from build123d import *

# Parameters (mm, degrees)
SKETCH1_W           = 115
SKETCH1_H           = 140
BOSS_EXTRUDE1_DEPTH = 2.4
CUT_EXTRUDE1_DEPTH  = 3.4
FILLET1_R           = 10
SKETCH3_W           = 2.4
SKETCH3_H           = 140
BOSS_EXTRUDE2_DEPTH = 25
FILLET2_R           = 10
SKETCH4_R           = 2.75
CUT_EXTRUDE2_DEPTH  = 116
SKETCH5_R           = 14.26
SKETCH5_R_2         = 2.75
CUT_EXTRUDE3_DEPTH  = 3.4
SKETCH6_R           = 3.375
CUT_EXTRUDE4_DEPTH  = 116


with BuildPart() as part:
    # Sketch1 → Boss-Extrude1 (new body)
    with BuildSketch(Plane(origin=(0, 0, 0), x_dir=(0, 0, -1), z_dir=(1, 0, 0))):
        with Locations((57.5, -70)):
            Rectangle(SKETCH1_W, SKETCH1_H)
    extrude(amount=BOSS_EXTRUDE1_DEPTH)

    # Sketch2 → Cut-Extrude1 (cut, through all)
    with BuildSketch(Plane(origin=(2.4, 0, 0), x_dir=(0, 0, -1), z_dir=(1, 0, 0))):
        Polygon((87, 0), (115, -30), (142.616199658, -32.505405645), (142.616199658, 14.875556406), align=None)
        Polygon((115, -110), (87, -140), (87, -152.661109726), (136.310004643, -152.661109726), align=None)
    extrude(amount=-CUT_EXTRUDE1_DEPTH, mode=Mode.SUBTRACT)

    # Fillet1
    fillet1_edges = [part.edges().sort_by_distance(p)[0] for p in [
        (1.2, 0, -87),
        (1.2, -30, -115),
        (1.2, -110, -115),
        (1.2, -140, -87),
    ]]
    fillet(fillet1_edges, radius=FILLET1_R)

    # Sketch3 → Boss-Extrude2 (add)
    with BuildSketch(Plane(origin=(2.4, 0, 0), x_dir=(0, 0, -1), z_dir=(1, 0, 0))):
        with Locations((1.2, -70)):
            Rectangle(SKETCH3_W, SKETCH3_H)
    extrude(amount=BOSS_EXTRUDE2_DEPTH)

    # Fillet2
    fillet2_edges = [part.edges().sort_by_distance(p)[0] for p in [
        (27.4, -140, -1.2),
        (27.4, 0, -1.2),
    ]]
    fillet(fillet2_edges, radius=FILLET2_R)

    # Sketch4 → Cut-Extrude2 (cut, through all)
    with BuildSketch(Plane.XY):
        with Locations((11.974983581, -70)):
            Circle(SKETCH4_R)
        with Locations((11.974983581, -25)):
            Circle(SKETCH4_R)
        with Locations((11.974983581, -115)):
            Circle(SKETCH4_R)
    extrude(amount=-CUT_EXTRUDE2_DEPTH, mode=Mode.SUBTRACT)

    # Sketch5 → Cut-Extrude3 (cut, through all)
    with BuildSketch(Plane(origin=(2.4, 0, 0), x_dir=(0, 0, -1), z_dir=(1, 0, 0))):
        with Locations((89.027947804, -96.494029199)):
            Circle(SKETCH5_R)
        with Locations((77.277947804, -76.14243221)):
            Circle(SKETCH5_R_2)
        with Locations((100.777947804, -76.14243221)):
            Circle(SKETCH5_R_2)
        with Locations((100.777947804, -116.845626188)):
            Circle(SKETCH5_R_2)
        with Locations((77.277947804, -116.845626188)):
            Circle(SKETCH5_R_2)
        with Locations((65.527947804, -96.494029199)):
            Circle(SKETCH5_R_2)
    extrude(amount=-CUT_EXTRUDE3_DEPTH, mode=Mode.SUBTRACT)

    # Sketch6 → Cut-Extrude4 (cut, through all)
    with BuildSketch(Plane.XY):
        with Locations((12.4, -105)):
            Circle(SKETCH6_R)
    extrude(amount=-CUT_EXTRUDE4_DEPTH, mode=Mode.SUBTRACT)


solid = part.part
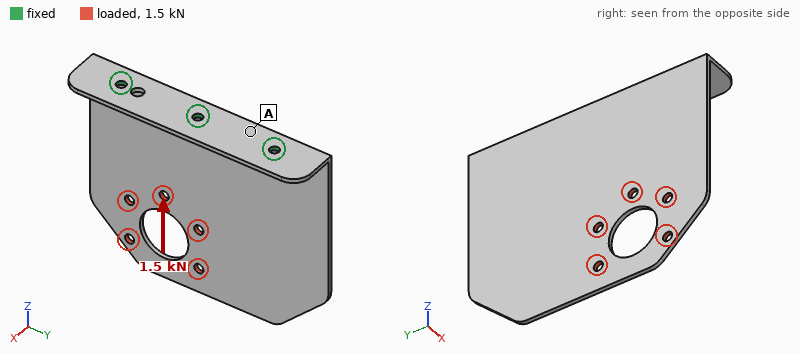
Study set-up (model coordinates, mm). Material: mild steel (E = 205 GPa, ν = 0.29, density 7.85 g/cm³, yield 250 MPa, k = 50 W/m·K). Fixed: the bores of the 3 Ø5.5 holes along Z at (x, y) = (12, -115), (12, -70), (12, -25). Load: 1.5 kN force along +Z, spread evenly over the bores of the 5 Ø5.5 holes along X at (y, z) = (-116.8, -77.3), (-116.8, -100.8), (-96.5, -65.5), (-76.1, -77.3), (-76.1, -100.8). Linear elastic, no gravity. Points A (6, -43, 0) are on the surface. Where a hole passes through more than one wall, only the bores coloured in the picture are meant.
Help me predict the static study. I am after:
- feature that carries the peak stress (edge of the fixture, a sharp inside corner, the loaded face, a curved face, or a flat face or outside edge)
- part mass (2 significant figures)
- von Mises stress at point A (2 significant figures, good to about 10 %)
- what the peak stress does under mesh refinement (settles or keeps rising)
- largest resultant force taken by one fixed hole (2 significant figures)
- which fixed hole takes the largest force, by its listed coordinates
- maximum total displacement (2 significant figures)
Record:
edge of the fixture
340 g
21 MPa
keeps rising
920 N
(12, -115)
0.40 mm
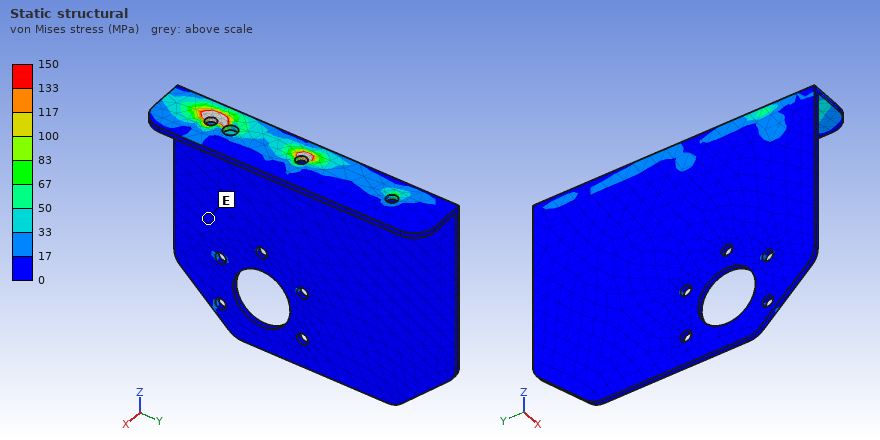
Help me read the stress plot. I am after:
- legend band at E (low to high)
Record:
0 to 17 MPa
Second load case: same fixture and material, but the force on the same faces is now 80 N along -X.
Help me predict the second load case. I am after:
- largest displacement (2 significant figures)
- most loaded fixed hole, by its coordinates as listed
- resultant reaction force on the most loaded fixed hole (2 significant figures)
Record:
1.1 mm
(12, -70)
51 N
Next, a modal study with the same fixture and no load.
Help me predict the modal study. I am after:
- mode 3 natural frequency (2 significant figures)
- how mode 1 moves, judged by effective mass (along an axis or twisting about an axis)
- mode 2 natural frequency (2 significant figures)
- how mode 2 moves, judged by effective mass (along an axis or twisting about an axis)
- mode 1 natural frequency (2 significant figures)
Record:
800 Hz
along X
360 Hz
twisting about Z
150 Hz
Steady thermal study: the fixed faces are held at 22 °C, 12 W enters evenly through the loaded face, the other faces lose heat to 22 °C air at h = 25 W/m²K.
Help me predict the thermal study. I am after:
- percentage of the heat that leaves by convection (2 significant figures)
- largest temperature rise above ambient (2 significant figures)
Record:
82 %
42 K
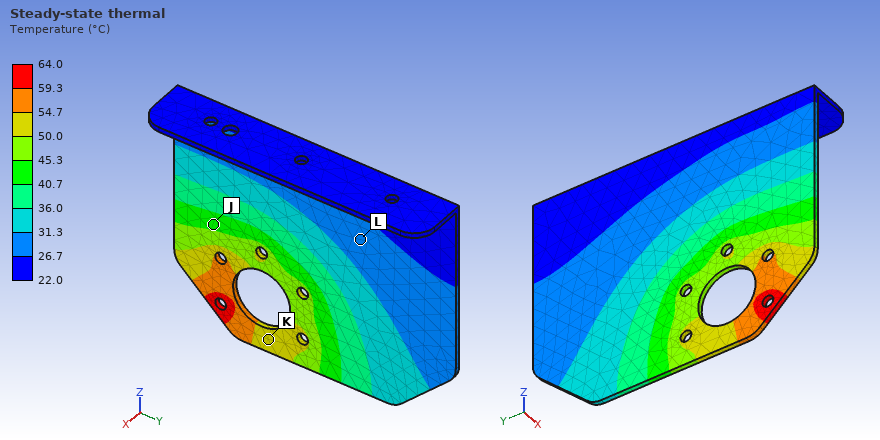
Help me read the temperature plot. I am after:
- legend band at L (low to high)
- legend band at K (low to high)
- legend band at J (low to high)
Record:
26.7 to 31.3 °C
50.0 to 54.7 °C
40.7 to 45.3 °C
